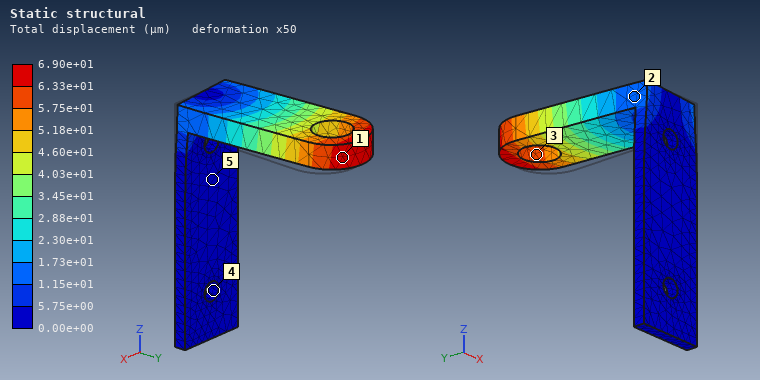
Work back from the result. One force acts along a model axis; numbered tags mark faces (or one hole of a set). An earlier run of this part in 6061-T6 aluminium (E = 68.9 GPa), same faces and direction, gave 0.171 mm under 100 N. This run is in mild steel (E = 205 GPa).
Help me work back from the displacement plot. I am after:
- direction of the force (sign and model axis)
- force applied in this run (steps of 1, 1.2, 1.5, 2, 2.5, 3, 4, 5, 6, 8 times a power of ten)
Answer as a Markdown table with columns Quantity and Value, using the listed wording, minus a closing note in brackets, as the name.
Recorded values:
| Quantity | Value |
|---|---|
| direction of the force | -X |
| force applied in this run | 120 N |
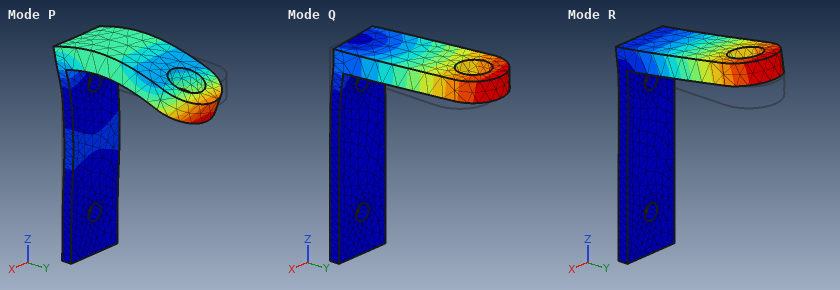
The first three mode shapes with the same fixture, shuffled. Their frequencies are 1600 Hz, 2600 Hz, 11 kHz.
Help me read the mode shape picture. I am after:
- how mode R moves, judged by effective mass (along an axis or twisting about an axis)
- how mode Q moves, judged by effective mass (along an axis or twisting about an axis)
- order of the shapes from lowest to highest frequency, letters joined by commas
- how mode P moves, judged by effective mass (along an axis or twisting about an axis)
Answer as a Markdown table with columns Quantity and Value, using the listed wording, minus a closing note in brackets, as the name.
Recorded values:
| Quantity | Value |
|---|---|
| how mode R moves, judged by effective mass | along Z |
| how mode Q moves, judged by effective mass | along X |
| order of the shapes from lowest to highest frequency, letters joined by commas | R, Q, P |
| how mode P moves, judged by effective mass | along Y |
